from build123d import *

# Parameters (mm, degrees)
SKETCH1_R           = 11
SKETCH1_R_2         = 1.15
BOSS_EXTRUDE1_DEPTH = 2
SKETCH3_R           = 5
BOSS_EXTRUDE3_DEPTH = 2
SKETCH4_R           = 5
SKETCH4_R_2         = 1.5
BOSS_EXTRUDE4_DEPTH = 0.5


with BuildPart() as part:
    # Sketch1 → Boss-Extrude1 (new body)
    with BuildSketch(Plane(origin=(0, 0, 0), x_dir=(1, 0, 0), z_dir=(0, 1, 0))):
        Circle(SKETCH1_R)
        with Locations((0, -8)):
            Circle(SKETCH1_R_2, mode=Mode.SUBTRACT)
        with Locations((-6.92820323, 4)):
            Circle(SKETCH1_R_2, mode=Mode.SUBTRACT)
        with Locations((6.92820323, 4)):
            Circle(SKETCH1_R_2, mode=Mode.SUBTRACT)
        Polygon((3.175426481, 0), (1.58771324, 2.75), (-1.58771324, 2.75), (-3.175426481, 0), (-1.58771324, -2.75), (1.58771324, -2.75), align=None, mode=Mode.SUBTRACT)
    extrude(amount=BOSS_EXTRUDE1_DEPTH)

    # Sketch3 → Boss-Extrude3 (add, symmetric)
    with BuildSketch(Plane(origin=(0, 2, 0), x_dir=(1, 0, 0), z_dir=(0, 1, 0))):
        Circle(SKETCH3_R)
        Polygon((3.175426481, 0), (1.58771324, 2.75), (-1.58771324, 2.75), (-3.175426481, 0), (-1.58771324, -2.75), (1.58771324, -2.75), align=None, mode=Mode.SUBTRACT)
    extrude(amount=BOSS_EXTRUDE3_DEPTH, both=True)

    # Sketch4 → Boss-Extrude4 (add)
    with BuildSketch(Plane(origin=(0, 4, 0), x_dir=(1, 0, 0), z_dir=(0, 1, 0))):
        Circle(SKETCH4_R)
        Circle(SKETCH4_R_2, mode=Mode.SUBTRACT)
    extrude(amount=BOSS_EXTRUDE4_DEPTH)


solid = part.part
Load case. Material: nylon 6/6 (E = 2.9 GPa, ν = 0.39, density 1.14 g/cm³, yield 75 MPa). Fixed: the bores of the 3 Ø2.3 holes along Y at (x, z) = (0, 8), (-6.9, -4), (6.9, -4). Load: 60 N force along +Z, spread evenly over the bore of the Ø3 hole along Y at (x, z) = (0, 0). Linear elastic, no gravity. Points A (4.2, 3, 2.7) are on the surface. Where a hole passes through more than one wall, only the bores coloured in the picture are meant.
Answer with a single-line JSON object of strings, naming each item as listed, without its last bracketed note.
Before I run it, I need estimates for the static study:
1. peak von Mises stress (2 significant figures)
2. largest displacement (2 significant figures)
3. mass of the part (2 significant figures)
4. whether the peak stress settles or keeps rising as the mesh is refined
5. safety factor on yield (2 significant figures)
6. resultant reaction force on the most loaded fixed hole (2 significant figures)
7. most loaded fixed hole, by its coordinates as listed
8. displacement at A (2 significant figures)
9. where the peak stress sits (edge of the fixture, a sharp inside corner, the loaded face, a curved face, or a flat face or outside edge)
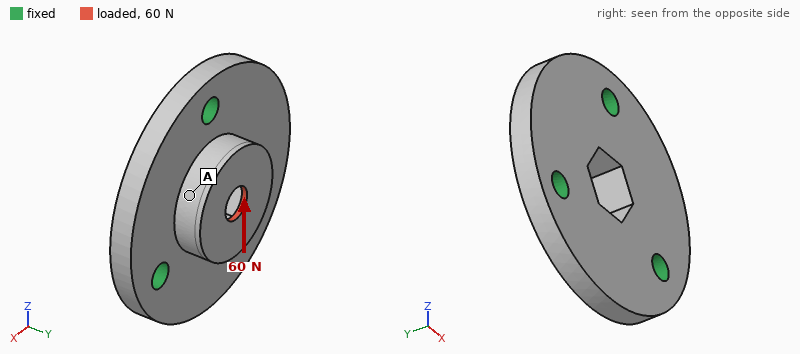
{"peak von Mises stress": "23 MPa", "largest displacement": "27 µm", "mass of the part": "0.94 g", "whether the peak stress settles or keeps rising as the mesh is refined": "settles", "safety factor on yield": "3.2", "resultant reaction force on the most loaded fixed hole": "27 N", "most loaded fixed hole, by its coordinates as listed": "(0, 8)", "displacement at A": "8.6 µm", "where the peak stress sits": "the loaded face"}
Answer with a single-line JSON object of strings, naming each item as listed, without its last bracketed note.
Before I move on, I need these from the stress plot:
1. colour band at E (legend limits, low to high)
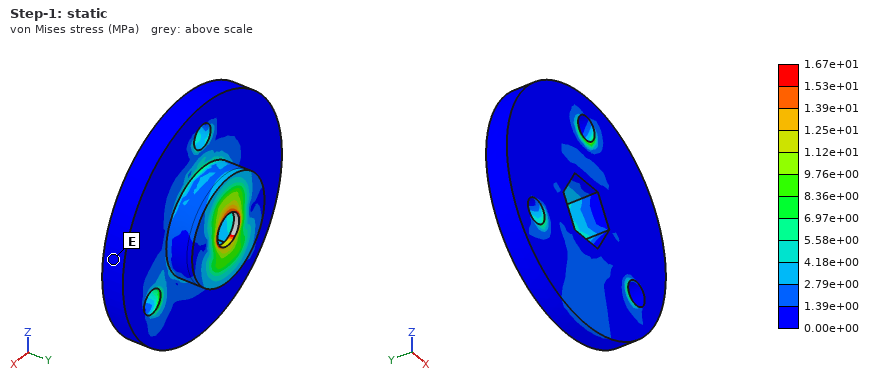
{"colour band at E": "0.00e+00 to 1.39e+00 MPa"}
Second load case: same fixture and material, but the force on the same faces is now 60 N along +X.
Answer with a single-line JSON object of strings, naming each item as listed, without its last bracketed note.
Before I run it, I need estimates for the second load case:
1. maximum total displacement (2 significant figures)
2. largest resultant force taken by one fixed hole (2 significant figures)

{"maximum total displacement": "26 µm", "largest resultant force taken by one fixed hole": "25 N"}
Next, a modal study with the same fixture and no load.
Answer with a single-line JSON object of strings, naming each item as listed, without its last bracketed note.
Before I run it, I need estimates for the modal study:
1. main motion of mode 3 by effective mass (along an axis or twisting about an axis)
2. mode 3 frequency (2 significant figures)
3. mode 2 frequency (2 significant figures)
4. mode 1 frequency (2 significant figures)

{"main motion of mode 3 by effective mass": "along Y", "mode 3 frequency": "12 kHz", "mode 2 frequency": "11 kHz", "mode 1 frequency": "11 kHz"}
